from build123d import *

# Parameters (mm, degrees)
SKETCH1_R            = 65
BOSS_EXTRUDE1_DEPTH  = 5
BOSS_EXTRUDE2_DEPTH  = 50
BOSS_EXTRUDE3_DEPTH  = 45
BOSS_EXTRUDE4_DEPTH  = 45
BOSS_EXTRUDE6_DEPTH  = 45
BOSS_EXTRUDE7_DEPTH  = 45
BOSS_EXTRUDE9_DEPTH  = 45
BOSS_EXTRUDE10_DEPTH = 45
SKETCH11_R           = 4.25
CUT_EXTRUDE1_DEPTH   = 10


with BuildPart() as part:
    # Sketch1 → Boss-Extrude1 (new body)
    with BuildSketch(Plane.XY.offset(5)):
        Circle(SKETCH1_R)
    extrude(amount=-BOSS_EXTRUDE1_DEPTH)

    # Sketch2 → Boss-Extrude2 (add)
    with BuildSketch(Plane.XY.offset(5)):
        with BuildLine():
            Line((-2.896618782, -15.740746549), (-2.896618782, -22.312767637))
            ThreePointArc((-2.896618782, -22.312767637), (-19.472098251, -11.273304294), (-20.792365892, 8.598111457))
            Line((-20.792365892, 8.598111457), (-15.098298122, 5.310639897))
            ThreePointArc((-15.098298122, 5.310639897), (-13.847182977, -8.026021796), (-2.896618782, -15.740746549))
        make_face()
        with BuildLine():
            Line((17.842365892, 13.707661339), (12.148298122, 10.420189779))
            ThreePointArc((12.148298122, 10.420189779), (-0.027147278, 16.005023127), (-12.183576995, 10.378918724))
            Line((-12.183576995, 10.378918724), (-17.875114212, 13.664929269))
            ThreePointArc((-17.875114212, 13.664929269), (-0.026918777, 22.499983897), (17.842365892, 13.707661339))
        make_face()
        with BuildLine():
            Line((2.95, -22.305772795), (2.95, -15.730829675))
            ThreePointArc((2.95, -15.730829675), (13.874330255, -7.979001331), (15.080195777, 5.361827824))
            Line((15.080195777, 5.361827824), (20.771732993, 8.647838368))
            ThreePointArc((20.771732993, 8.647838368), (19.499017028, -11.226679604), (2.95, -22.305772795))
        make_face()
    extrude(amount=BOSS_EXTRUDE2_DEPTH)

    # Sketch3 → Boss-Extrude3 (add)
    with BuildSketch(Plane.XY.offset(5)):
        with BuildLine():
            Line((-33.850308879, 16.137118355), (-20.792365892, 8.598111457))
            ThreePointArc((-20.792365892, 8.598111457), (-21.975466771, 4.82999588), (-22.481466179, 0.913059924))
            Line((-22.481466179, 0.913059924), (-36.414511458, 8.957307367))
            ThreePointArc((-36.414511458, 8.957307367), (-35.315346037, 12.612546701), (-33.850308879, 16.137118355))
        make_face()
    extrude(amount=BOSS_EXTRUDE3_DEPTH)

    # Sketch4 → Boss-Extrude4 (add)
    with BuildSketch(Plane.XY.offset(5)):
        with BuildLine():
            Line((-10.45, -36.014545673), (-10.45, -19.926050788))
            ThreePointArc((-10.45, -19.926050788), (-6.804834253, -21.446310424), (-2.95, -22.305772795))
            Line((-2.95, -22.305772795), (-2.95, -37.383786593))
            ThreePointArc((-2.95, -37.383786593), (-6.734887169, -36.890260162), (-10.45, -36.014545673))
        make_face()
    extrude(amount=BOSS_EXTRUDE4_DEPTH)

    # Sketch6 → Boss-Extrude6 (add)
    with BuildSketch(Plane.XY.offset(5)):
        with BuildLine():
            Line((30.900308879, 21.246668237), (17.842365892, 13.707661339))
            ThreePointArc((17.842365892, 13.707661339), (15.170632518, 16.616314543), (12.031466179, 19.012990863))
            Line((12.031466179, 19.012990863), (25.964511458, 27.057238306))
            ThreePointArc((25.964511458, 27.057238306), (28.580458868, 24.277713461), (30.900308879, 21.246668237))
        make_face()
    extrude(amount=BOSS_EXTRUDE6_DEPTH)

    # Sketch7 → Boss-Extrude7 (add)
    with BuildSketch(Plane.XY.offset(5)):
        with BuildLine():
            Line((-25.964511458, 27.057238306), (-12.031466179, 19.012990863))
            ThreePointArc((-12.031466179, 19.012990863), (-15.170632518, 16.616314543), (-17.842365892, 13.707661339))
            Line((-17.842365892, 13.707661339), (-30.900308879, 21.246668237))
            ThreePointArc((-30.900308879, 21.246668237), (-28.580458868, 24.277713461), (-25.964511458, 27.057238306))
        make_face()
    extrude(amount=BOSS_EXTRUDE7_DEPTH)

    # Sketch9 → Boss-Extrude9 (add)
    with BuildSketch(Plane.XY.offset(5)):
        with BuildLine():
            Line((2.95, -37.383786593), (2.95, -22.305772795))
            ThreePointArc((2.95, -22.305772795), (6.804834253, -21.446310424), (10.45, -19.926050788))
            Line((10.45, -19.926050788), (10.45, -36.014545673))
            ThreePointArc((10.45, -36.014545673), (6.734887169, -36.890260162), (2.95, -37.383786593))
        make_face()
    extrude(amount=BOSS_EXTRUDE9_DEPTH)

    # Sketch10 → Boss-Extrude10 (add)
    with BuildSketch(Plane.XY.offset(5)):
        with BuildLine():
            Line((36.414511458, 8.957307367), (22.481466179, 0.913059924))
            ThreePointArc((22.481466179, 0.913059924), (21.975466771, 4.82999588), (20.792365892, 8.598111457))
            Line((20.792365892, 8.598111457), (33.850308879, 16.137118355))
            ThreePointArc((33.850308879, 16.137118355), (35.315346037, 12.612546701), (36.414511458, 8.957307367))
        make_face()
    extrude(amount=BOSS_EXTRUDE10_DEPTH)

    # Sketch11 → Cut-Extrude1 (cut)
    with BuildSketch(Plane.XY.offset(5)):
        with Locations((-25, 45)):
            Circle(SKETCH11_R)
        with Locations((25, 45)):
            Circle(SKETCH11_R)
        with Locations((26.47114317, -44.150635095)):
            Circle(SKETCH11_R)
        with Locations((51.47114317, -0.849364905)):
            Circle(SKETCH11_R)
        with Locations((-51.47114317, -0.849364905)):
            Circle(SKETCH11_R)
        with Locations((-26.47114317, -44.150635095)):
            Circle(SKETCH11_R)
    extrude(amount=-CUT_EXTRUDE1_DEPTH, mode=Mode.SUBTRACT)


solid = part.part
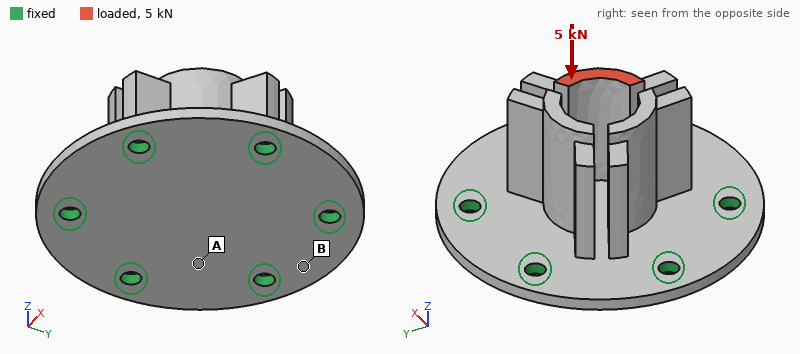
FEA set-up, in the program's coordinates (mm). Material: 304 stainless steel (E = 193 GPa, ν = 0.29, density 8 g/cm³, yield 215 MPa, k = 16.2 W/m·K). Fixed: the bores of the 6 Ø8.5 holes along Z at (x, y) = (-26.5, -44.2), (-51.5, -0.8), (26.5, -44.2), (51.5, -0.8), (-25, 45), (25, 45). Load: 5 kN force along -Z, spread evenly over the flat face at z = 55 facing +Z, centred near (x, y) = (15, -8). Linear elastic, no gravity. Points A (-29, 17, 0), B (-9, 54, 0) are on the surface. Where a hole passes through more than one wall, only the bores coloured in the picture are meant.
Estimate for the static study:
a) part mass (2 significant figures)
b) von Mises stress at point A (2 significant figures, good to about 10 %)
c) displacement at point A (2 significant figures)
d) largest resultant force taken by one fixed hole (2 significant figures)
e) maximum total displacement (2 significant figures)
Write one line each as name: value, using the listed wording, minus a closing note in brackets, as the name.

part mass: 1.0 kg
von Mises stress at point A: 35 MPa
displacement at point A: 12 µm
largest resultant force taken by one fixed hole: 1.4 kN
maximum total displacement: 77 µm
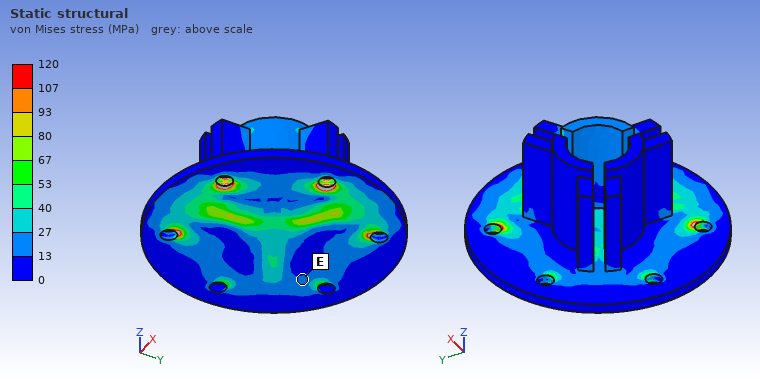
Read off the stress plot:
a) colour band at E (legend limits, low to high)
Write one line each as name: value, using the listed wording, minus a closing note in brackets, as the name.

colour band at E: 13 to 27 MPa
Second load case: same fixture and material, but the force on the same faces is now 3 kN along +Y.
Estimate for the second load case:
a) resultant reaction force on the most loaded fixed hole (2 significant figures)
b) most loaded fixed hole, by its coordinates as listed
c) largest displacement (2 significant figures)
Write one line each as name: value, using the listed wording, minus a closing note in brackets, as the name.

resultant reaction force on the most loaded fixed hole: 2.1 kN
most loaded fixed hole, by its coordinates as listed: (26.5, -44.2)
largest displacement: 0.20 mm
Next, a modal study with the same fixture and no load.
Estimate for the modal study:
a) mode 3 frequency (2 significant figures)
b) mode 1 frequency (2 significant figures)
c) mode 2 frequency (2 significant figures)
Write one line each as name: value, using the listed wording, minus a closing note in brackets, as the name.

mode 3 frequency: 2600 Hz
mode 1 frequency: 1600 Hz
mode 2 frequency: 2600 Hz
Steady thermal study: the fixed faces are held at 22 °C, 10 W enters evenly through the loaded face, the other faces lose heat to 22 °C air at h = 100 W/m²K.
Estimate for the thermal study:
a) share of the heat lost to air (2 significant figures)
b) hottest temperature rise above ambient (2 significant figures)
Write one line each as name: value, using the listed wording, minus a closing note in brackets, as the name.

share of the heat lost to air: 96 %
hottest temperature rise above ambient: 48 K
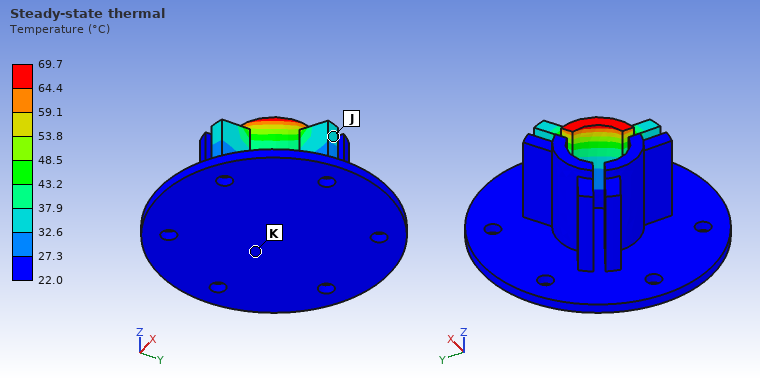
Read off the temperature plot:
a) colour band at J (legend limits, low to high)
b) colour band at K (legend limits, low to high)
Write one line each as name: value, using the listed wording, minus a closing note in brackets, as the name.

colour band at J: 32.6 to 37.9 °C
colour band at K: 22.0 to 27.3 °C
